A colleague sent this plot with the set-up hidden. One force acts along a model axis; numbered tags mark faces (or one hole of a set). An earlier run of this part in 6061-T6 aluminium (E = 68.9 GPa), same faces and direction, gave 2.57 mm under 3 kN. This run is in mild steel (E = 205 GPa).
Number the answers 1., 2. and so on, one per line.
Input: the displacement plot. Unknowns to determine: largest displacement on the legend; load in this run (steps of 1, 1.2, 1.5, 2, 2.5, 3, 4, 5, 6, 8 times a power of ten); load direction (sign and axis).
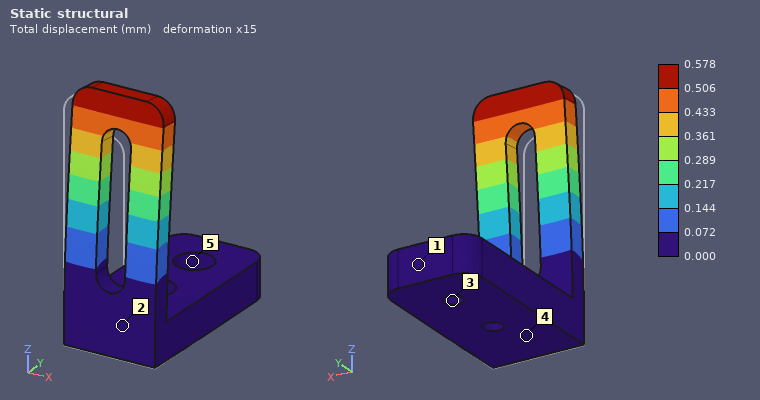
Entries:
1. 0.578 mm
2. 2 kN
3. +Y
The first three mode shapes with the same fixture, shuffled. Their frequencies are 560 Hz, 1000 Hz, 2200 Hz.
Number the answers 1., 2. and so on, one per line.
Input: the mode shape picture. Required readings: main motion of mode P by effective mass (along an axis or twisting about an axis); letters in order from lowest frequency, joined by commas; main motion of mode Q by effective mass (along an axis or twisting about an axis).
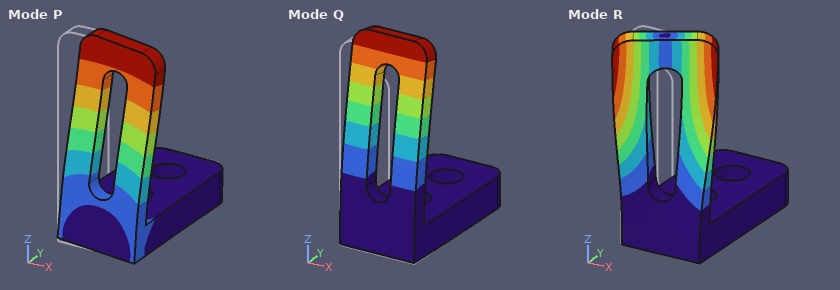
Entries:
1. along X
2. Q, P, R
3. along Y
